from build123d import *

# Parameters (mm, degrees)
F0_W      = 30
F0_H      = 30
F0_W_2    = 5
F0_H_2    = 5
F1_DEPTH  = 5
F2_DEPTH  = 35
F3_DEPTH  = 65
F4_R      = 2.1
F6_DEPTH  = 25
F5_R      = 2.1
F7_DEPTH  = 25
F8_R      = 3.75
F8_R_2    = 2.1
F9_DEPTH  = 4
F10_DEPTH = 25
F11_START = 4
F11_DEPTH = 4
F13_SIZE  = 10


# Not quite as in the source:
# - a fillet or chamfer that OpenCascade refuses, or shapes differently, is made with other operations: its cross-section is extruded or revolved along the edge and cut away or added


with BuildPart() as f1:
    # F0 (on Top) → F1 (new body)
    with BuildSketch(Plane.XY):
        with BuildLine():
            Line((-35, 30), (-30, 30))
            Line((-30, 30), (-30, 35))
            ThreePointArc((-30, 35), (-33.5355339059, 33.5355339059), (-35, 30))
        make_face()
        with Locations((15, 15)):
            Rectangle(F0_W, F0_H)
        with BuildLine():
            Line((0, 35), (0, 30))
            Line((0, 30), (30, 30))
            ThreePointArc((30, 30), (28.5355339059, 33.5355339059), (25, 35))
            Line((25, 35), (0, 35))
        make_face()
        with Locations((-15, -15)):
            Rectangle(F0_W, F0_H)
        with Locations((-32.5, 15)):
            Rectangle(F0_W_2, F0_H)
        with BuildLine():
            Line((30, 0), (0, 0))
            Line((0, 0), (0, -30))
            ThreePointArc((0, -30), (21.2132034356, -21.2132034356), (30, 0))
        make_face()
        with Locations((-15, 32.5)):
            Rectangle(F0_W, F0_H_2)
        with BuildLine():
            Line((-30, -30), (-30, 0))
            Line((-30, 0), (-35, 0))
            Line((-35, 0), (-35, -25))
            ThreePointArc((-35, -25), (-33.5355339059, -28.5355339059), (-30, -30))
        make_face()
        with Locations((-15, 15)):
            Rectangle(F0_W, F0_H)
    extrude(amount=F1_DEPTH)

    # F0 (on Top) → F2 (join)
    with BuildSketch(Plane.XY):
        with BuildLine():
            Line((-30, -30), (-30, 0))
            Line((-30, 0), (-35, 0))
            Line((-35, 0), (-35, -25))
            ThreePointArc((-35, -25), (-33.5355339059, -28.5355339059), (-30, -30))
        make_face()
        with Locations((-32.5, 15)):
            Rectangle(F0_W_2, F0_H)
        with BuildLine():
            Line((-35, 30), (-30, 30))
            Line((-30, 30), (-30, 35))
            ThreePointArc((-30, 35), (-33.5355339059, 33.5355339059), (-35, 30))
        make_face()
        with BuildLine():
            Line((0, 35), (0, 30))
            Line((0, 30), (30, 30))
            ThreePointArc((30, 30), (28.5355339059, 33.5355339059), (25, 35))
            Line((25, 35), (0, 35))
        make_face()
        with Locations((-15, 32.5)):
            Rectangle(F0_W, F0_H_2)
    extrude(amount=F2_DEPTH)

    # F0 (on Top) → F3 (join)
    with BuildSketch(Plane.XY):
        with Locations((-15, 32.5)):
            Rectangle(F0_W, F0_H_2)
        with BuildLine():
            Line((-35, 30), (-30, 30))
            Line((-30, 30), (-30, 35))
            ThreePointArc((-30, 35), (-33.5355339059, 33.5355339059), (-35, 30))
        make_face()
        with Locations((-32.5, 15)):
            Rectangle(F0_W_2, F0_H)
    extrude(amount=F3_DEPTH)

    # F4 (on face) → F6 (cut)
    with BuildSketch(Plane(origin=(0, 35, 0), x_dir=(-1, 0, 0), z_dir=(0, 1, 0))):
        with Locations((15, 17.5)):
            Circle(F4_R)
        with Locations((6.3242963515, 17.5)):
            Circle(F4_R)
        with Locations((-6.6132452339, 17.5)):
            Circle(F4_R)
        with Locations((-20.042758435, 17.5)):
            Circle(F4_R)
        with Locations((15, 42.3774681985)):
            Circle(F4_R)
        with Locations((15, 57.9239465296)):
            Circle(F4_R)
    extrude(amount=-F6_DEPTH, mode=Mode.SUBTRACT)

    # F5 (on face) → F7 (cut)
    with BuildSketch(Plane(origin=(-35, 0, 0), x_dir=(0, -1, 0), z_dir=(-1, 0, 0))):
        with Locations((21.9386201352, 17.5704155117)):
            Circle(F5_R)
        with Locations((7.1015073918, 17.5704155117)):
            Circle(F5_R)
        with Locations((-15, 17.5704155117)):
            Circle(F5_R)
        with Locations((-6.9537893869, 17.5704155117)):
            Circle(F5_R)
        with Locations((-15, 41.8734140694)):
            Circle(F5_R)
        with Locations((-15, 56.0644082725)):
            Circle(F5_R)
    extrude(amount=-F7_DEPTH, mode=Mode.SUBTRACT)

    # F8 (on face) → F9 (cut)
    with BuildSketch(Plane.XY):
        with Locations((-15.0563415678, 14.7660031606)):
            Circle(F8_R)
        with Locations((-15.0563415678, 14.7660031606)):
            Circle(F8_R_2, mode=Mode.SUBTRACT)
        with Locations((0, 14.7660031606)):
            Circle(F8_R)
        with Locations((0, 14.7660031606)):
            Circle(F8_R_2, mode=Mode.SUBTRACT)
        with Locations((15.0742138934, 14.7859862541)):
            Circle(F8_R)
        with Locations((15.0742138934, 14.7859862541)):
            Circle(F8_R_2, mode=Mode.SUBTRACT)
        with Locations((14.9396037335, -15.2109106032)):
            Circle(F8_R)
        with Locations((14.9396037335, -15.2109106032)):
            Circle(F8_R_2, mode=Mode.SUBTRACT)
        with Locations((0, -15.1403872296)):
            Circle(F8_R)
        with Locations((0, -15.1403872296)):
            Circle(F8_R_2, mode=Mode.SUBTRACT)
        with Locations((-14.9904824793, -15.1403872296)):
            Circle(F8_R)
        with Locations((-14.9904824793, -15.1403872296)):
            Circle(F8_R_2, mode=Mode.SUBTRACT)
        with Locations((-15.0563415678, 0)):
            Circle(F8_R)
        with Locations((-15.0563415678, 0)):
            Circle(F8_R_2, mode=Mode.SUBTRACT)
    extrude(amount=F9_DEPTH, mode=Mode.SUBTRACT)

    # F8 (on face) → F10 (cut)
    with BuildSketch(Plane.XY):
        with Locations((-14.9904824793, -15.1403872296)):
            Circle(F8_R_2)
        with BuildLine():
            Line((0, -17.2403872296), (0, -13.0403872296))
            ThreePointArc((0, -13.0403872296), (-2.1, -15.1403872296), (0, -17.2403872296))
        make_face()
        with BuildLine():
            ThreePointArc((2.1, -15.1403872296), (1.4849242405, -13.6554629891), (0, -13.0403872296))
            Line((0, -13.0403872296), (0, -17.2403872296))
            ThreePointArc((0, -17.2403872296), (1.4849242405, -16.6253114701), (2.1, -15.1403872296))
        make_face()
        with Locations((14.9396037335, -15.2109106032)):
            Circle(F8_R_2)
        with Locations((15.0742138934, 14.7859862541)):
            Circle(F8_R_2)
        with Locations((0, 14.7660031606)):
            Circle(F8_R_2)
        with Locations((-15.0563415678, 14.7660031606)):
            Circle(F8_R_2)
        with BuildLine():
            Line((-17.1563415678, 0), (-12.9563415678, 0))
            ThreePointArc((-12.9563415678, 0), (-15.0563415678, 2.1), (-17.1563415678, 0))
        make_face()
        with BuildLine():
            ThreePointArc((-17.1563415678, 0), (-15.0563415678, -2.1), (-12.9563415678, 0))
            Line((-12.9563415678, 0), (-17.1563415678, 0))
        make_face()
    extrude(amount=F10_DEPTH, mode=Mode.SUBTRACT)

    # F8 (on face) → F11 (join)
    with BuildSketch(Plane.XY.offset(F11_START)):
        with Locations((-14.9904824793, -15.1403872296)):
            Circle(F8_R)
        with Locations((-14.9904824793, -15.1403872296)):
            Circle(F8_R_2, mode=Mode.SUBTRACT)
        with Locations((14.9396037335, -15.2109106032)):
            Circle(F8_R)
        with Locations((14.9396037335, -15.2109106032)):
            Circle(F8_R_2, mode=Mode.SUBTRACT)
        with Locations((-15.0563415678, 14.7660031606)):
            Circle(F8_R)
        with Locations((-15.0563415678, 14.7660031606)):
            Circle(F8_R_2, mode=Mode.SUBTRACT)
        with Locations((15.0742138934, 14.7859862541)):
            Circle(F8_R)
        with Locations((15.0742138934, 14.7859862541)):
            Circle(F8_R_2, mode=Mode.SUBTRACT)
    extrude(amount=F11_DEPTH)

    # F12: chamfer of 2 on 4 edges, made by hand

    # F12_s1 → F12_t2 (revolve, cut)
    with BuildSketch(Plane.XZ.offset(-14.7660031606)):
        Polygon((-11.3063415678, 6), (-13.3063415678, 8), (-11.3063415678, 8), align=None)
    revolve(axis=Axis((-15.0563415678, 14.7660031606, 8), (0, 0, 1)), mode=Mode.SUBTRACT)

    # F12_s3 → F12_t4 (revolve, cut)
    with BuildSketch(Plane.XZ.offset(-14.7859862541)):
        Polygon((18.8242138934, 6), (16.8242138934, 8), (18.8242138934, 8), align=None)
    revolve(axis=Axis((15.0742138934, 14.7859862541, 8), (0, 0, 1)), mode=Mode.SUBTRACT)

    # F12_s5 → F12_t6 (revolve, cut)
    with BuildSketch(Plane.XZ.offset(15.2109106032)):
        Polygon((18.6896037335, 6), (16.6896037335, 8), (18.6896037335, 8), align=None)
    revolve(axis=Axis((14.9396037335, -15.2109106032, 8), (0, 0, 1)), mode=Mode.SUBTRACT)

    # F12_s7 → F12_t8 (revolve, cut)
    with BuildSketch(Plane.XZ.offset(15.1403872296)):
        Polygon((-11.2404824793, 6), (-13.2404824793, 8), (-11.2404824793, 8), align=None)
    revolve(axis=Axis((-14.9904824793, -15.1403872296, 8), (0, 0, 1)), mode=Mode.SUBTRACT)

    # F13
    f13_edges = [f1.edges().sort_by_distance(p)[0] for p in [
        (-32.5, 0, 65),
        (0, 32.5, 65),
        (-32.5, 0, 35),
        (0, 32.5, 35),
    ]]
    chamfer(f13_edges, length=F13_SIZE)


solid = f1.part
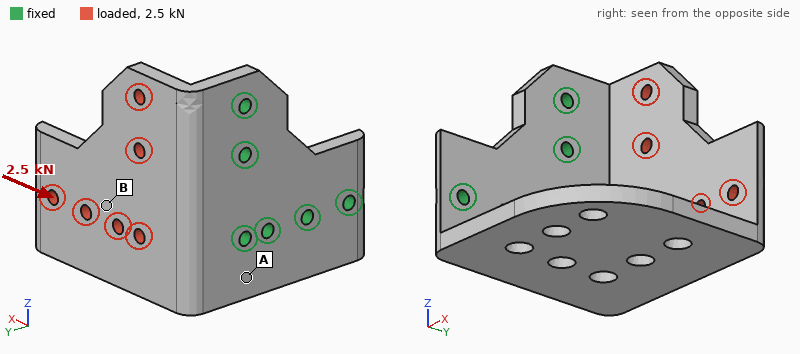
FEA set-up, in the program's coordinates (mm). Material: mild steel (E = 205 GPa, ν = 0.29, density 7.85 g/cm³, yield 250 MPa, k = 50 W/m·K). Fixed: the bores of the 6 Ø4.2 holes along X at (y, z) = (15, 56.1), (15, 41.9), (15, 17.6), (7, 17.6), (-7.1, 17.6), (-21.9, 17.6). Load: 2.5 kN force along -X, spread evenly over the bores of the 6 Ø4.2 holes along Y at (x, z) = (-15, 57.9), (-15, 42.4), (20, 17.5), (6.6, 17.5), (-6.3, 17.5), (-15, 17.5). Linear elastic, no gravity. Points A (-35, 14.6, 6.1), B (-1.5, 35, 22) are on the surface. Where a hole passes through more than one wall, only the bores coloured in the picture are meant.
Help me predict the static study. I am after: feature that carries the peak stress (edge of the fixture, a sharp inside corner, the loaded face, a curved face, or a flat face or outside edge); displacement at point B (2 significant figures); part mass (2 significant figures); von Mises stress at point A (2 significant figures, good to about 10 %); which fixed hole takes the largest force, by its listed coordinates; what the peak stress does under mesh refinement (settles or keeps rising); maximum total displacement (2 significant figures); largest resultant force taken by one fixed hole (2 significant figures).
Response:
edge of the fixture
34 µm
360 g
33 MPa
(15, 17.6)
keeps rising
55 µm
1.9 kN
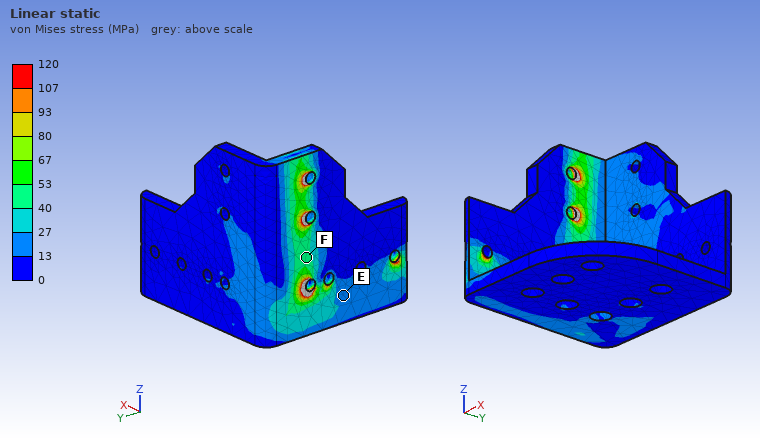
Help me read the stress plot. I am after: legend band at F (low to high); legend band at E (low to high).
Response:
40 to 53 MPa
13 to 27 MPa
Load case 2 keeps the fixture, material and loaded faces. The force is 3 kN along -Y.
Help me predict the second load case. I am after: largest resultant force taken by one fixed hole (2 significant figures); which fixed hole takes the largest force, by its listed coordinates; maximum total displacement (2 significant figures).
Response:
2.2 kN
(15, 17.6)
0.21 mm
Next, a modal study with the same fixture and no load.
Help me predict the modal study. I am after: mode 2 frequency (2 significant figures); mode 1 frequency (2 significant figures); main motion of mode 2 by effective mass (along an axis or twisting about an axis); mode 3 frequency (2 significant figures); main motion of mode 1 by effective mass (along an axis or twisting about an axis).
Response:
1900 Hz
1600 Hz
along Y
3300 Hz
along Z
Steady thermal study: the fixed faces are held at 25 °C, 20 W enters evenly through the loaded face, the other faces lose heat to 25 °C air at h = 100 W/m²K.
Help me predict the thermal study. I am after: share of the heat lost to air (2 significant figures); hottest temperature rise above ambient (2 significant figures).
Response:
67 %
20 K
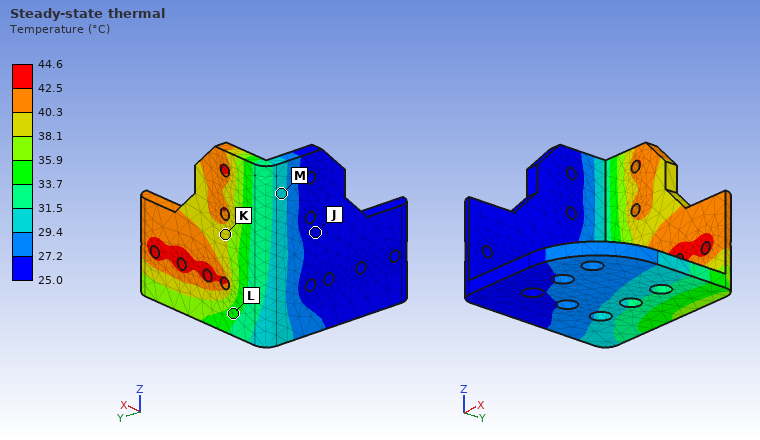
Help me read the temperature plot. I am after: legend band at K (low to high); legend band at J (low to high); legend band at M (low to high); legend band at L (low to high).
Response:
38.1 to 40.3 °C
25.0 to 27.2 °C
29.4 to 31.5 °C
33.7 to 35.9 °C
